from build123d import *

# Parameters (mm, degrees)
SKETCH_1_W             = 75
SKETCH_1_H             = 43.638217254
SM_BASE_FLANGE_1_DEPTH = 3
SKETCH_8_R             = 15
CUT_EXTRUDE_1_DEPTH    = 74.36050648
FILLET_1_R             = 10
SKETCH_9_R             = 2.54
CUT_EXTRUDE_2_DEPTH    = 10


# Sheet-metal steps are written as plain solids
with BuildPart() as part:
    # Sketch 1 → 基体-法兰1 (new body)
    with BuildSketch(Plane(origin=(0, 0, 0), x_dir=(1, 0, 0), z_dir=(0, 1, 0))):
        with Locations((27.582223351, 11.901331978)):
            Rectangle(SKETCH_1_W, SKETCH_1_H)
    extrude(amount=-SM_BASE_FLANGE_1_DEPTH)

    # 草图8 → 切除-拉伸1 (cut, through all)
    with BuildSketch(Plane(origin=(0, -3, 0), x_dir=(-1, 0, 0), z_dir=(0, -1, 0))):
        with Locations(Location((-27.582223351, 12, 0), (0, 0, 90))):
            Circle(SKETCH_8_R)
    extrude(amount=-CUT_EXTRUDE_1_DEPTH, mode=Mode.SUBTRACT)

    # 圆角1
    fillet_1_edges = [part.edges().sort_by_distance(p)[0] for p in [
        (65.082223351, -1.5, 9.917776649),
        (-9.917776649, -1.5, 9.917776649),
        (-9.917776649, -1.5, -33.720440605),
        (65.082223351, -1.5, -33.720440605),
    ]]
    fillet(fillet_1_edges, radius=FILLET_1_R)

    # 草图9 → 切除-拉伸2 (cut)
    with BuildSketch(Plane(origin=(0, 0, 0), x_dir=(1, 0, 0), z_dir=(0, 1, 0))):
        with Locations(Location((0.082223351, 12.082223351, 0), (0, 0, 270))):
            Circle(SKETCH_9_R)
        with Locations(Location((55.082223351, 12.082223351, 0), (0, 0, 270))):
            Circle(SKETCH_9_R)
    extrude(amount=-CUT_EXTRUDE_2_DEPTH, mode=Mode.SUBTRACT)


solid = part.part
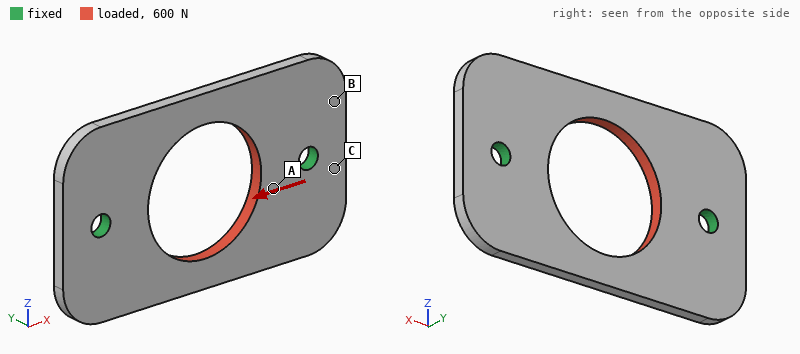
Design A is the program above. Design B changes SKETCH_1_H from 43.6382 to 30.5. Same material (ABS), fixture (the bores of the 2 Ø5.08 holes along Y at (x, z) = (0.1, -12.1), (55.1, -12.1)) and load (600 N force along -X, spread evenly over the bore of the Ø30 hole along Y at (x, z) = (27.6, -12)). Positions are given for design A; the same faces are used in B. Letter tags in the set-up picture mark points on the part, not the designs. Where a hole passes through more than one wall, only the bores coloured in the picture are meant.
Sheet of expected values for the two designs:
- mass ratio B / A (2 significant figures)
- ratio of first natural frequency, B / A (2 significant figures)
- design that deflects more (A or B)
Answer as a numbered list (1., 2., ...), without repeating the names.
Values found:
1. 0.60
2. 1.9
3. B
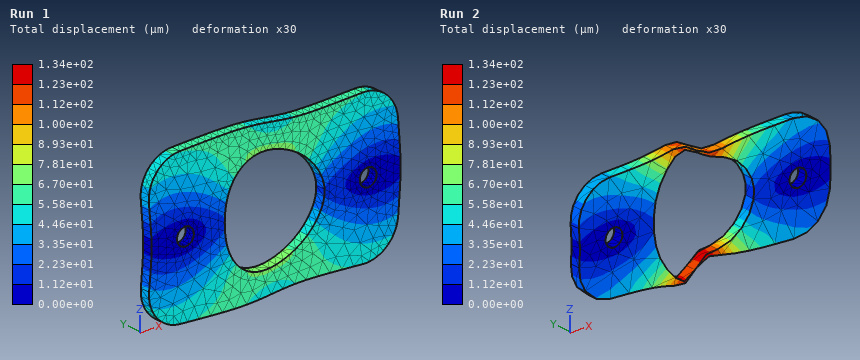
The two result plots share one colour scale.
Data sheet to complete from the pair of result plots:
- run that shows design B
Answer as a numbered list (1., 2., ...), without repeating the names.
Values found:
1. Run 2
